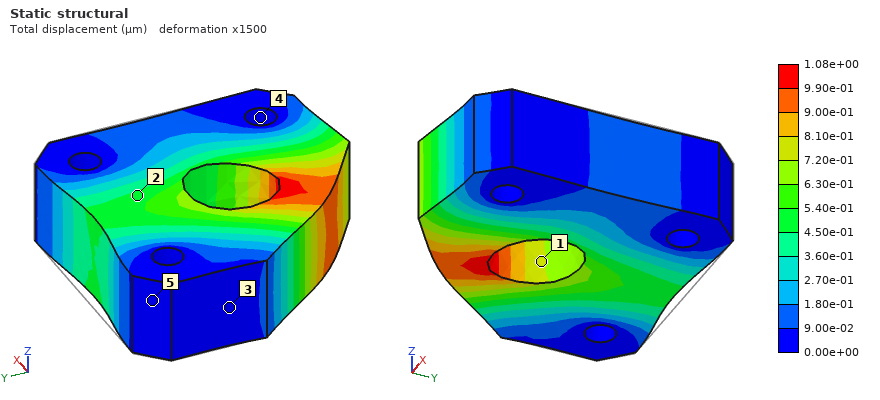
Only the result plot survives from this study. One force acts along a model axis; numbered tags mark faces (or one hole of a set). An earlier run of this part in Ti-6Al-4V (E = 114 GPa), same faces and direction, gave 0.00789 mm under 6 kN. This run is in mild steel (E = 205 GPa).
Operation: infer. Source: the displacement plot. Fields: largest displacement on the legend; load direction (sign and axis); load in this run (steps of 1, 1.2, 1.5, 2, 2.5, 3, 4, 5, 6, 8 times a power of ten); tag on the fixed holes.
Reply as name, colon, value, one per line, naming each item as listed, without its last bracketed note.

largest displacement on the legend: 1.08e+00 µm
load direction: -Y
load in this run: 1.5 kN
tag on the fixed holes: 4
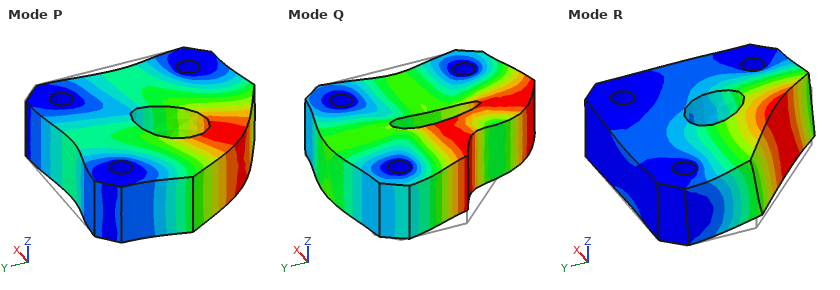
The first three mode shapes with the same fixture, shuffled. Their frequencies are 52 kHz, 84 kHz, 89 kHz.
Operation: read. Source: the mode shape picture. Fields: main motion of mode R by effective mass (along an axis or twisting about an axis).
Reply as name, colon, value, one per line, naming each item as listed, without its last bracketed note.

main motion of mode R by effective mass: along Z
